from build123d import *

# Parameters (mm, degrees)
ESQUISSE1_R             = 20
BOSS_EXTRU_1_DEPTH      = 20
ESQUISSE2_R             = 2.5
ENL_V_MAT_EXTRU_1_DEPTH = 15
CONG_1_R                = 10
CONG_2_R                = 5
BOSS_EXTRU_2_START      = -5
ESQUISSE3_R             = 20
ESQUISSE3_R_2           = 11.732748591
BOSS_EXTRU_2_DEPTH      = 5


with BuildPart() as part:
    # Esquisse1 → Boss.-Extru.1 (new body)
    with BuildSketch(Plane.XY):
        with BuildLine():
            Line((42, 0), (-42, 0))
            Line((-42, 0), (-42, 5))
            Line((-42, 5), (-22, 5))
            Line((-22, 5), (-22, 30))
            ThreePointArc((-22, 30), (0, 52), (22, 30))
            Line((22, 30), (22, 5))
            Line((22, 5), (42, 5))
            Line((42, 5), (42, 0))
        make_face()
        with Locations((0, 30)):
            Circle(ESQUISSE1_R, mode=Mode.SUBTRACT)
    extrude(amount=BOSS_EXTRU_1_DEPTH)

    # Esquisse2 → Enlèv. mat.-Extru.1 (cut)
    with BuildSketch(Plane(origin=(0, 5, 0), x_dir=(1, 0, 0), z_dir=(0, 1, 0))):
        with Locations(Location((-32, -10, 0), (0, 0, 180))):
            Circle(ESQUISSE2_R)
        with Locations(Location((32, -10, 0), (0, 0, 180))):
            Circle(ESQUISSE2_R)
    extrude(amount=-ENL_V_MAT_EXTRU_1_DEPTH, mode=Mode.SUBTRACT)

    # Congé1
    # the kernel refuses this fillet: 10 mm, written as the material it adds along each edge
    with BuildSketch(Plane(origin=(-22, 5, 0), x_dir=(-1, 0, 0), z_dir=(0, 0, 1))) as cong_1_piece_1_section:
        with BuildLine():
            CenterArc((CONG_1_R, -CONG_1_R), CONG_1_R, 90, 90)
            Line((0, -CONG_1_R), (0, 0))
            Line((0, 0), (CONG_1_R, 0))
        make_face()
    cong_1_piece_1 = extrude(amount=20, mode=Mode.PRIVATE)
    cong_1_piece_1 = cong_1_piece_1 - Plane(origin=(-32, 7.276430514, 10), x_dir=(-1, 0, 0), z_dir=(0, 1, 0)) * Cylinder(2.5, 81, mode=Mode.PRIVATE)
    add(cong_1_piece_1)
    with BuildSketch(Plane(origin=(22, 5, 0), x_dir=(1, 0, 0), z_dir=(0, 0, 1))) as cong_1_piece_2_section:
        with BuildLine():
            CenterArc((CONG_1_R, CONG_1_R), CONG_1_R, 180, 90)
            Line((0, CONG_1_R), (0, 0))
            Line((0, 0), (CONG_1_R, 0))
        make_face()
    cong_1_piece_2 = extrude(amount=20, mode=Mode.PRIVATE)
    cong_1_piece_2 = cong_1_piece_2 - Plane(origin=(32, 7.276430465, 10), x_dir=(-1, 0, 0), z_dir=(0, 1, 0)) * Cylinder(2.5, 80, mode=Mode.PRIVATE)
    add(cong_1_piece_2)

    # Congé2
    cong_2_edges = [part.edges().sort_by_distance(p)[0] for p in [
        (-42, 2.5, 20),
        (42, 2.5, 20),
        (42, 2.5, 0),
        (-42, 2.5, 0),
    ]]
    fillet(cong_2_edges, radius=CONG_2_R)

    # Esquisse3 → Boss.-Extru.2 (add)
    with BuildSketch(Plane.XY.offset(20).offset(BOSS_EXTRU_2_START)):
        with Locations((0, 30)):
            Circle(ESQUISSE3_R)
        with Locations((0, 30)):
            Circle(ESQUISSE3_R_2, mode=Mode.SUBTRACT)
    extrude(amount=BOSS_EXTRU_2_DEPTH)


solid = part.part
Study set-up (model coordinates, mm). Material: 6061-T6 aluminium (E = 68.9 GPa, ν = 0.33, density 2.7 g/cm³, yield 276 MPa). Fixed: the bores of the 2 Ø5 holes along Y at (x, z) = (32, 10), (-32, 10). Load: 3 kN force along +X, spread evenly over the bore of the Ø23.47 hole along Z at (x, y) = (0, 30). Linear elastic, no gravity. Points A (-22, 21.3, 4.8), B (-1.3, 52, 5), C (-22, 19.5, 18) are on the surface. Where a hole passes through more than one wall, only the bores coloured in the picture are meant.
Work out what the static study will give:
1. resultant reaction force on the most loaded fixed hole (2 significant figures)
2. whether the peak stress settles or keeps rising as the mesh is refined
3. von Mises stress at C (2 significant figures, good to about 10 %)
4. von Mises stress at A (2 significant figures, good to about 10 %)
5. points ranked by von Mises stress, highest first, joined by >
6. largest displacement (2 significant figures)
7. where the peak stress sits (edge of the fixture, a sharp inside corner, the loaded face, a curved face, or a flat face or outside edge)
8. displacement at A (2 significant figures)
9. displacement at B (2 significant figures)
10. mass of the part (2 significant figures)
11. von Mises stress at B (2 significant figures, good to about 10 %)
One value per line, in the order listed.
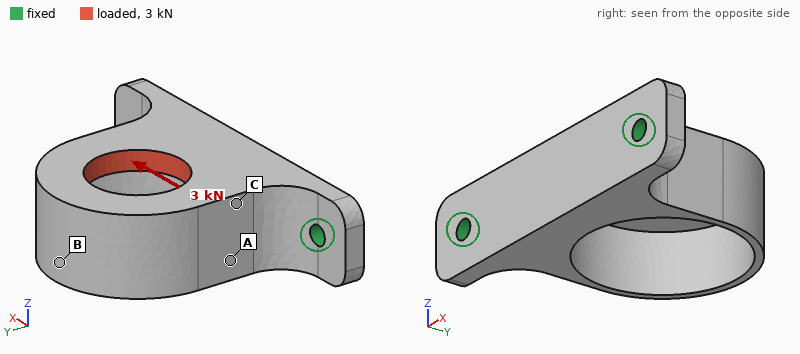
2.1 kN
keeps rising
45 MPa
28 MPa
C > A > B
94 µm
edge of the fixture
15 µm
80 µm
68 g
13 MPa
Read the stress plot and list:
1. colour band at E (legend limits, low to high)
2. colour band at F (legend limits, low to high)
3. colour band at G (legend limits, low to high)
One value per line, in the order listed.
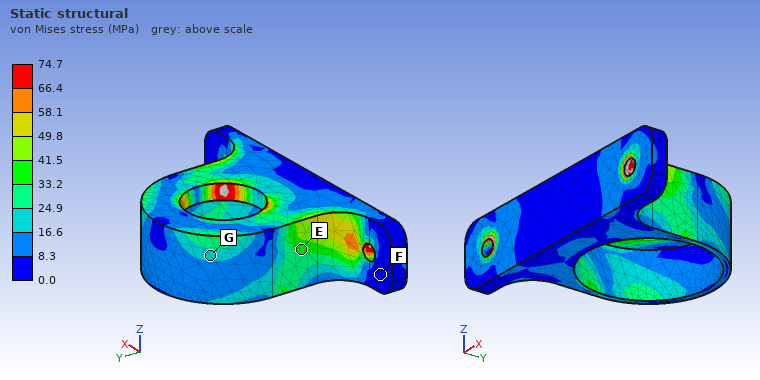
33.2 to 41.5 MPa
0.0 to 8.3 MPa
16.6 to 24.9 MPa
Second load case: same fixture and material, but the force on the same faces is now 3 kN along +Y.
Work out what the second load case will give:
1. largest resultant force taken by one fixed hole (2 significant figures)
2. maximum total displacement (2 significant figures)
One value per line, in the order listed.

1.9 kN
0.17 mm
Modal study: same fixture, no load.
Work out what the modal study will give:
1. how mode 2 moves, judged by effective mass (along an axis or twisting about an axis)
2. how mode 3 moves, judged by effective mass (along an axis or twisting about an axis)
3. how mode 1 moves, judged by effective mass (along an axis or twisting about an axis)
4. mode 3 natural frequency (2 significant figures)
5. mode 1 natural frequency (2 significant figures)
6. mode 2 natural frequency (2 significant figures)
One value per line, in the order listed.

along X
along Y
along Z
8100 Hz
2500 Hz
5600 Hz
